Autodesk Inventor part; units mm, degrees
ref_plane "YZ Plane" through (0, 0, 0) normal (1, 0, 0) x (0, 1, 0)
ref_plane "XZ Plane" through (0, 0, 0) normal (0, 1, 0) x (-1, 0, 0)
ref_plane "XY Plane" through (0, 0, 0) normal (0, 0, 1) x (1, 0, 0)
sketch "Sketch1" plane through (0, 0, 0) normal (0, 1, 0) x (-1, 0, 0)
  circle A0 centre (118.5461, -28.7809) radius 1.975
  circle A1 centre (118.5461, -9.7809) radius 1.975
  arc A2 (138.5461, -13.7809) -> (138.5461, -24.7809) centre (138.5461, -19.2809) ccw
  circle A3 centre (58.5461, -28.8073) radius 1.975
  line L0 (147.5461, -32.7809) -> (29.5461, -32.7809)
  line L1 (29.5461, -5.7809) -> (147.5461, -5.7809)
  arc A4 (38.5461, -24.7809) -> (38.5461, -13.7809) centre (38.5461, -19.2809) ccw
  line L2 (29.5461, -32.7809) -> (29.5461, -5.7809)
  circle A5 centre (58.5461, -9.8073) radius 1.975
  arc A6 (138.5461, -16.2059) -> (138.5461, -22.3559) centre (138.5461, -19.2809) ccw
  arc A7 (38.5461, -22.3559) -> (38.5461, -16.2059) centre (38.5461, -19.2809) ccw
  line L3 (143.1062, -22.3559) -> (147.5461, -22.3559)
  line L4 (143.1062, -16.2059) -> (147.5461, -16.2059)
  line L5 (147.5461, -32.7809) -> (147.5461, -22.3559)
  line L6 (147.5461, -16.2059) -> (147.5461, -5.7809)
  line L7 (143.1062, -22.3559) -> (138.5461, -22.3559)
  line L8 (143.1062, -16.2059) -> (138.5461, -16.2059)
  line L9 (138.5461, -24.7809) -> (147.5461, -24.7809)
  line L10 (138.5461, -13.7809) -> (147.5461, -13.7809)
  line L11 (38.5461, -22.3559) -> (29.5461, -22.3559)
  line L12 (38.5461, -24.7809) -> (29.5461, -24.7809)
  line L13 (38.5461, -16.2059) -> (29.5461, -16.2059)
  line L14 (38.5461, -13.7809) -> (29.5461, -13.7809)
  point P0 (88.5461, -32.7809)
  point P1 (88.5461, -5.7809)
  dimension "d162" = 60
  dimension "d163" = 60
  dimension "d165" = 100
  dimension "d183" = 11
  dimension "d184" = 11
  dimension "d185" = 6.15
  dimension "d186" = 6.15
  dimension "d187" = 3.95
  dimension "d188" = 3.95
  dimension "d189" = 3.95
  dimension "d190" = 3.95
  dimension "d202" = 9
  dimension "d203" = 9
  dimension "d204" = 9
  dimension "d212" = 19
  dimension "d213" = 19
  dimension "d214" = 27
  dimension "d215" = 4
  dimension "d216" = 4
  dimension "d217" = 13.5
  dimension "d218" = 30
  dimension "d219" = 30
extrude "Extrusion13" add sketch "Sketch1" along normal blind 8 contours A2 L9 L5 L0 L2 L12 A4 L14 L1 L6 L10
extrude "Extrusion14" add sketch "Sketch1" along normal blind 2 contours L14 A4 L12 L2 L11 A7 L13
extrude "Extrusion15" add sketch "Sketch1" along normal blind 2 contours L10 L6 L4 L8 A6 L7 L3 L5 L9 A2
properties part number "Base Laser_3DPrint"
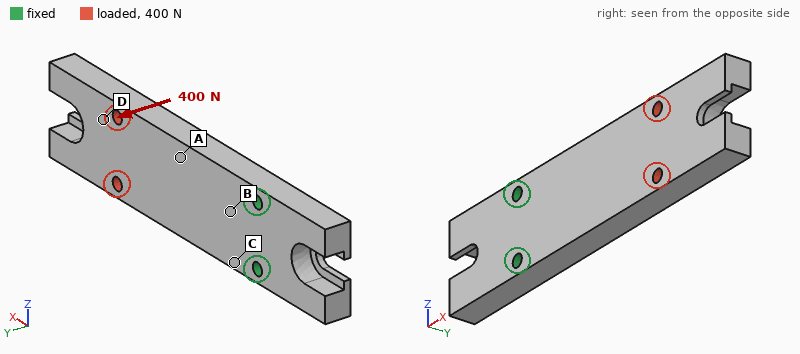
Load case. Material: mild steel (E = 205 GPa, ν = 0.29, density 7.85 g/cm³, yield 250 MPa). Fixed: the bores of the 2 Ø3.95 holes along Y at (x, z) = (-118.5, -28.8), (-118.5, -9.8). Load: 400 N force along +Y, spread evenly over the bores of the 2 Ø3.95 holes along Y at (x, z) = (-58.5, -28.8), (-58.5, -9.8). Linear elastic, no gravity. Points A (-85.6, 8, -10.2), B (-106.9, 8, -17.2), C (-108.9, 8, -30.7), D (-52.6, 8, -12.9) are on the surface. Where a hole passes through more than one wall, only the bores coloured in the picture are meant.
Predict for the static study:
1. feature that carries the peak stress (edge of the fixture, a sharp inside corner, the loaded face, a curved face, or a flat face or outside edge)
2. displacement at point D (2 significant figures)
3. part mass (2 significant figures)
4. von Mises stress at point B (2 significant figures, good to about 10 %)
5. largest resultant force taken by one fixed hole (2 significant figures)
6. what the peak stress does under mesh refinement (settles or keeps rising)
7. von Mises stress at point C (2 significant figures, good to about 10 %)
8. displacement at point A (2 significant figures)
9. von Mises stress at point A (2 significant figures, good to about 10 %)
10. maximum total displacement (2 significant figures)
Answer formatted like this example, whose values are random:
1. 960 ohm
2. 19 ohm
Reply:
1. edge of the fixture
2. 0.14 mm
3. 180 g
4. 63 MPa
5. 200 N
6. keeps rising
7. 73 MPa
8. 0.048 mm
9. 38 MPa
10. 0.21 mm
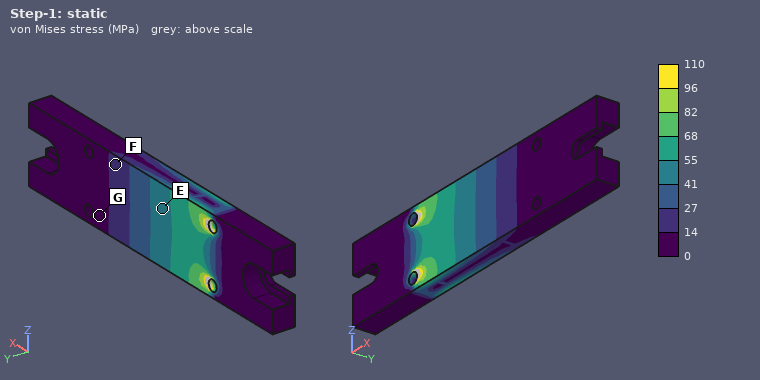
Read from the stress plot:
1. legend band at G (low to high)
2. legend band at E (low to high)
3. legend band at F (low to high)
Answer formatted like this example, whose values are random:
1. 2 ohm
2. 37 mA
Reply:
1. 0 to 14 MPa
2. 41 to 55 MPa
3. 14 to 27 MPa
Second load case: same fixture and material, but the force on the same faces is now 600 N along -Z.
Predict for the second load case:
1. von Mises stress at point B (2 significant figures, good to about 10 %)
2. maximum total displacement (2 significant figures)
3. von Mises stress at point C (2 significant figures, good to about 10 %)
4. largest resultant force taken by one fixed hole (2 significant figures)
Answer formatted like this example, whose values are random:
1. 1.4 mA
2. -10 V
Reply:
1. 8.5 MPa
2. 30 µm
3. 26 MPa
4. 1.8 kN
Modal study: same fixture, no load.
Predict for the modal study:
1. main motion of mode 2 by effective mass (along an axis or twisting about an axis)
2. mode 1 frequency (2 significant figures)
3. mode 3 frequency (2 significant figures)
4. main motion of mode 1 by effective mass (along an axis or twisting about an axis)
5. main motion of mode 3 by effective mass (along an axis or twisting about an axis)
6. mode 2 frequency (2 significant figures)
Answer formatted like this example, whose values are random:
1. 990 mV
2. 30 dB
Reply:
1. along Z
2. 910 Hz
3. 4900 Hz
4. along Y
5. twisting about X
6. 2900 Hz
